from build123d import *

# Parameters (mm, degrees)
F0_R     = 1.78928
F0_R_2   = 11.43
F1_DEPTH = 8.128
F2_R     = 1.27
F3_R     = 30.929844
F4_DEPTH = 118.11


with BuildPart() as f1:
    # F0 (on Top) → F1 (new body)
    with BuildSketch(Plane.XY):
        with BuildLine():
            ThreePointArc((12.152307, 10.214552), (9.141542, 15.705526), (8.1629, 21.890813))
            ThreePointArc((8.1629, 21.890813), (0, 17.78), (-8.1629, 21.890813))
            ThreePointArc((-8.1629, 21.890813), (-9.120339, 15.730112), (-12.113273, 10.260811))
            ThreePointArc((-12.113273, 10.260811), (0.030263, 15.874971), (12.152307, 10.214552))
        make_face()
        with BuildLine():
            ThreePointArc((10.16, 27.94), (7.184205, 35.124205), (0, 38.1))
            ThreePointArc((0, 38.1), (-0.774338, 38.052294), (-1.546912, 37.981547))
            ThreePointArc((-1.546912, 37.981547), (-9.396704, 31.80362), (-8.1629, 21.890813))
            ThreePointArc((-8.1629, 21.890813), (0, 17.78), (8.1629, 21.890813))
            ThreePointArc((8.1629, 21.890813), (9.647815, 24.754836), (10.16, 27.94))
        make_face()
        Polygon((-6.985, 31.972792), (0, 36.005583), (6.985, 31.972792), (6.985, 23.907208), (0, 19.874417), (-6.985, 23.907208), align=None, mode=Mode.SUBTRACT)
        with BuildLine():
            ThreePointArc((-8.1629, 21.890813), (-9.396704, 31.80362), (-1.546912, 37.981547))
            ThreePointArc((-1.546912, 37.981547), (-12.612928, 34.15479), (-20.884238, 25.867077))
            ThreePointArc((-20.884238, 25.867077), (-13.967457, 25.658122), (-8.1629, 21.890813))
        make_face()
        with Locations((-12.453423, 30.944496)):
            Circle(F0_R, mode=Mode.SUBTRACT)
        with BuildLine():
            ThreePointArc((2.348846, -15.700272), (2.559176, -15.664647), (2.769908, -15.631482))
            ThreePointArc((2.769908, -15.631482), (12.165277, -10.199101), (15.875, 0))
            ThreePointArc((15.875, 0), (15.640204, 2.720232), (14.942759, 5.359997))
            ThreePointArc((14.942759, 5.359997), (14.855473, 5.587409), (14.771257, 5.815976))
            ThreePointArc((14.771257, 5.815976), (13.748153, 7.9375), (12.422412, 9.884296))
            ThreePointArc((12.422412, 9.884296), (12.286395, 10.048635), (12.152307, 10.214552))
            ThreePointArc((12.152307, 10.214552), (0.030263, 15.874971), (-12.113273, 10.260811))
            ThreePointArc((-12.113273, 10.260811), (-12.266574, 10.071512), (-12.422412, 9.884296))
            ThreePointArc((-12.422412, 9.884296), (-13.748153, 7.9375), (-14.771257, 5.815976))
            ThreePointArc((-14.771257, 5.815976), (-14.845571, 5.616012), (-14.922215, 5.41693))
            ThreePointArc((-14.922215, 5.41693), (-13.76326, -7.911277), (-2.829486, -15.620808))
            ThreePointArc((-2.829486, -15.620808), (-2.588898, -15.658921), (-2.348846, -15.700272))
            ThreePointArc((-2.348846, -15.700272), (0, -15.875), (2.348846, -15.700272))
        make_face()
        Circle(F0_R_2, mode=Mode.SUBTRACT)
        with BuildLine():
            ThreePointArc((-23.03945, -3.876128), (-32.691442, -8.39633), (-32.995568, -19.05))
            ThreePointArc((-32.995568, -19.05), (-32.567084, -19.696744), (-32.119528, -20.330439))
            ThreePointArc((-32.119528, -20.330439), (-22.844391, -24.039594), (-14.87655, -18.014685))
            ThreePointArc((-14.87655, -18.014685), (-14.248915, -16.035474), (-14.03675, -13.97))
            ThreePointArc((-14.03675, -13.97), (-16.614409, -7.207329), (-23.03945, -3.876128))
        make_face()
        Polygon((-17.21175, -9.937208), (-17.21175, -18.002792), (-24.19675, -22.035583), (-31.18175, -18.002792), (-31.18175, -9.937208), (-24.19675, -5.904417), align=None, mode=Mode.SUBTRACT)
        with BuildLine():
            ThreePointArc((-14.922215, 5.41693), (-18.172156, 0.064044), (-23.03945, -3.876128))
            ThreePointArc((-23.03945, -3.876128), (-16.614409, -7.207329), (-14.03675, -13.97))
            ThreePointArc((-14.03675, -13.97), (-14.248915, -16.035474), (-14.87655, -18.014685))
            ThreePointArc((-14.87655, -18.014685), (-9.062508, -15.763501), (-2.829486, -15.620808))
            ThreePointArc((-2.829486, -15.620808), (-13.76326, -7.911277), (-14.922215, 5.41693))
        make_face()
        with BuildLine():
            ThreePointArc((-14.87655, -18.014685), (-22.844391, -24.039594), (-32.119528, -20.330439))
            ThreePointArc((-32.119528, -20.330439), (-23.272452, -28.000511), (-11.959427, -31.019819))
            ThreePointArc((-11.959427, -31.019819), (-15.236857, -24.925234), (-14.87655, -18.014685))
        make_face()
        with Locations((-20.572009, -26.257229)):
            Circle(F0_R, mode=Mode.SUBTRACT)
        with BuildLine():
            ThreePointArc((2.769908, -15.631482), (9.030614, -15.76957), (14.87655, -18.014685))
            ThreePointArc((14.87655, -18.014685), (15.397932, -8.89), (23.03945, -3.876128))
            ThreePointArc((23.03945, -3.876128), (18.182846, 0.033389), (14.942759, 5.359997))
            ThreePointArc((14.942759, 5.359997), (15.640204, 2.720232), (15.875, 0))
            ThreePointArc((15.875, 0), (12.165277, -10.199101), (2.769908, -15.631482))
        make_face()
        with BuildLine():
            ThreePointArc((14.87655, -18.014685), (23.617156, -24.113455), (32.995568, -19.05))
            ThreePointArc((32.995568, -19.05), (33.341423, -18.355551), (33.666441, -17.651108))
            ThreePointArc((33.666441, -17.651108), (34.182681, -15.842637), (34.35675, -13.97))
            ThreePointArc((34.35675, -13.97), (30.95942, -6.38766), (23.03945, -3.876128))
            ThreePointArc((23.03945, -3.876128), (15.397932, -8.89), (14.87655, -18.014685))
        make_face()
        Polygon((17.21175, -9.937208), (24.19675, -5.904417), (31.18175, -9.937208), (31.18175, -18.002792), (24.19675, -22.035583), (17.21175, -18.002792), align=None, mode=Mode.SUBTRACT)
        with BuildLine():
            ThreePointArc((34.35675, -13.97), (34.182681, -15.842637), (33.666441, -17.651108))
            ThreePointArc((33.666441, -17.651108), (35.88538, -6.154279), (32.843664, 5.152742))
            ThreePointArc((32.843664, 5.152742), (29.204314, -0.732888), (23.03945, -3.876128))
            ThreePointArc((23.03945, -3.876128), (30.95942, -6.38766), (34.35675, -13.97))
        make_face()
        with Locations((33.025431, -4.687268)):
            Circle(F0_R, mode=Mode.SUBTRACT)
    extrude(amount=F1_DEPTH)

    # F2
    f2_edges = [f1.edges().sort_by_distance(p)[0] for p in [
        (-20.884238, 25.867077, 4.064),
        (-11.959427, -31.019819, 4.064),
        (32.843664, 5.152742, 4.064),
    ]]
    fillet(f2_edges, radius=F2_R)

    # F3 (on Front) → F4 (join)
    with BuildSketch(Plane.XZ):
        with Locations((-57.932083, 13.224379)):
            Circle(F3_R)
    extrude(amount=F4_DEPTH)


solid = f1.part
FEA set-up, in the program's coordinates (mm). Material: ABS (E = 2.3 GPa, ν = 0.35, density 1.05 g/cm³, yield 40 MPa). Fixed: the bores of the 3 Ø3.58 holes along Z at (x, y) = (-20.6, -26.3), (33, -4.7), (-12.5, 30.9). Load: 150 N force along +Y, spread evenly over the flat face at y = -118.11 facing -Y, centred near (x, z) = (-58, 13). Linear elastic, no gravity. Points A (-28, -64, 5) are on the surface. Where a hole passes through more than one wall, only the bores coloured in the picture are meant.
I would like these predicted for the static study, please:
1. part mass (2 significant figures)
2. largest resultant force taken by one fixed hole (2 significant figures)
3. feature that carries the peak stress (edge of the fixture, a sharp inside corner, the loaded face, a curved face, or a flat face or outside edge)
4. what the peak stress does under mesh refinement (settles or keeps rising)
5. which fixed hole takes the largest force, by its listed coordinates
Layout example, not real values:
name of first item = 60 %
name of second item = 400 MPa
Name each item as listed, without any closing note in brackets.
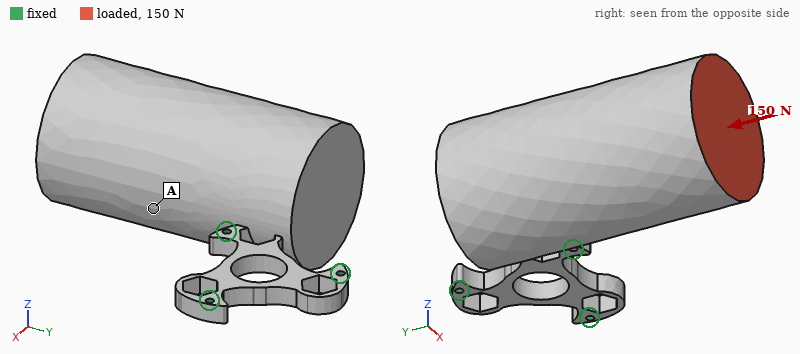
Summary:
part mass = 380 g
largest resultant force taken by one fixed hole = 240 N
feature that carries the peak stress = edge of the fixture
what the peak stress does under mesh refinement = keeps rising
which fixed hole takes the largest force, by its listed coordinates = (-20.6, -26.3)
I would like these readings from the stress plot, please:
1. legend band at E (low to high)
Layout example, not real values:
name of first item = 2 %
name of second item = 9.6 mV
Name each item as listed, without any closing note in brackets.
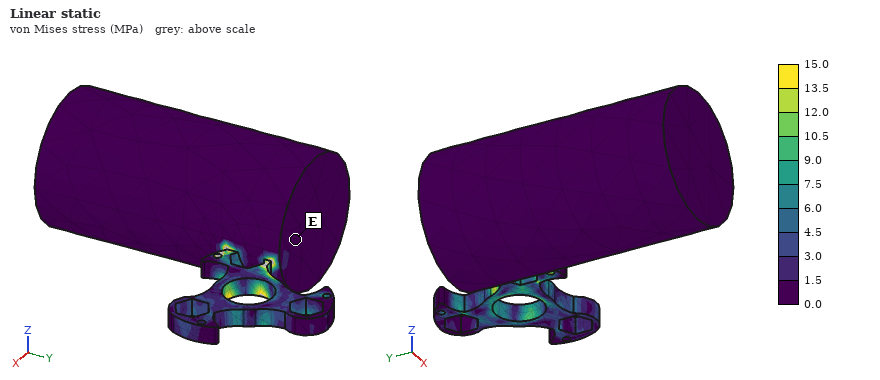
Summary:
legend band at E = 0.0 to 1.5 MPa
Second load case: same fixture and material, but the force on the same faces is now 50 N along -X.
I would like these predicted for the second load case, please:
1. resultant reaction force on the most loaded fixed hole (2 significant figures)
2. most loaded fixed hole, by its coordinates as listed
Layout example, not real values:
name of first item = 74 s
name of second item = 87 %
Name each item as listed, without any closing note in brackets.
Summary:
resultant reaction force on the most loaded fixed hole = 230 N
most loaded fixed hole, by its coordinates as listed = (-20.6, -26.3)
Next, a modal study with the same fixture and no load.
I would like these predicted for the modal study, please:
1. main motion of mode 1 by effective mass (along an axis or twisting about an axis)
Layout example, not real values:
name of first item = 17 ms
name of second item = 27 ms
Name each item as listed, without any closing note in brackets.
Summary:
main motion of mode 1 by effective mass = along Z
